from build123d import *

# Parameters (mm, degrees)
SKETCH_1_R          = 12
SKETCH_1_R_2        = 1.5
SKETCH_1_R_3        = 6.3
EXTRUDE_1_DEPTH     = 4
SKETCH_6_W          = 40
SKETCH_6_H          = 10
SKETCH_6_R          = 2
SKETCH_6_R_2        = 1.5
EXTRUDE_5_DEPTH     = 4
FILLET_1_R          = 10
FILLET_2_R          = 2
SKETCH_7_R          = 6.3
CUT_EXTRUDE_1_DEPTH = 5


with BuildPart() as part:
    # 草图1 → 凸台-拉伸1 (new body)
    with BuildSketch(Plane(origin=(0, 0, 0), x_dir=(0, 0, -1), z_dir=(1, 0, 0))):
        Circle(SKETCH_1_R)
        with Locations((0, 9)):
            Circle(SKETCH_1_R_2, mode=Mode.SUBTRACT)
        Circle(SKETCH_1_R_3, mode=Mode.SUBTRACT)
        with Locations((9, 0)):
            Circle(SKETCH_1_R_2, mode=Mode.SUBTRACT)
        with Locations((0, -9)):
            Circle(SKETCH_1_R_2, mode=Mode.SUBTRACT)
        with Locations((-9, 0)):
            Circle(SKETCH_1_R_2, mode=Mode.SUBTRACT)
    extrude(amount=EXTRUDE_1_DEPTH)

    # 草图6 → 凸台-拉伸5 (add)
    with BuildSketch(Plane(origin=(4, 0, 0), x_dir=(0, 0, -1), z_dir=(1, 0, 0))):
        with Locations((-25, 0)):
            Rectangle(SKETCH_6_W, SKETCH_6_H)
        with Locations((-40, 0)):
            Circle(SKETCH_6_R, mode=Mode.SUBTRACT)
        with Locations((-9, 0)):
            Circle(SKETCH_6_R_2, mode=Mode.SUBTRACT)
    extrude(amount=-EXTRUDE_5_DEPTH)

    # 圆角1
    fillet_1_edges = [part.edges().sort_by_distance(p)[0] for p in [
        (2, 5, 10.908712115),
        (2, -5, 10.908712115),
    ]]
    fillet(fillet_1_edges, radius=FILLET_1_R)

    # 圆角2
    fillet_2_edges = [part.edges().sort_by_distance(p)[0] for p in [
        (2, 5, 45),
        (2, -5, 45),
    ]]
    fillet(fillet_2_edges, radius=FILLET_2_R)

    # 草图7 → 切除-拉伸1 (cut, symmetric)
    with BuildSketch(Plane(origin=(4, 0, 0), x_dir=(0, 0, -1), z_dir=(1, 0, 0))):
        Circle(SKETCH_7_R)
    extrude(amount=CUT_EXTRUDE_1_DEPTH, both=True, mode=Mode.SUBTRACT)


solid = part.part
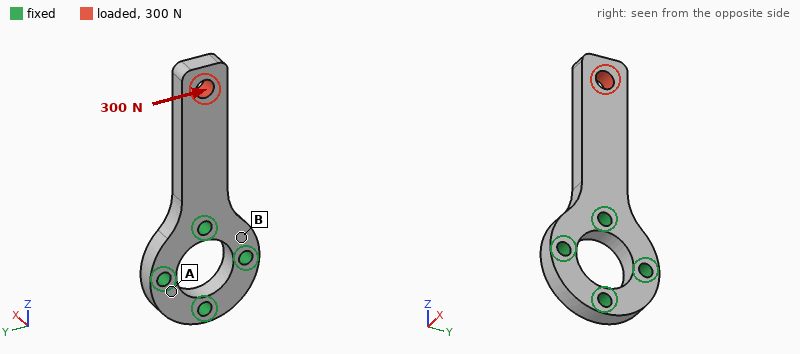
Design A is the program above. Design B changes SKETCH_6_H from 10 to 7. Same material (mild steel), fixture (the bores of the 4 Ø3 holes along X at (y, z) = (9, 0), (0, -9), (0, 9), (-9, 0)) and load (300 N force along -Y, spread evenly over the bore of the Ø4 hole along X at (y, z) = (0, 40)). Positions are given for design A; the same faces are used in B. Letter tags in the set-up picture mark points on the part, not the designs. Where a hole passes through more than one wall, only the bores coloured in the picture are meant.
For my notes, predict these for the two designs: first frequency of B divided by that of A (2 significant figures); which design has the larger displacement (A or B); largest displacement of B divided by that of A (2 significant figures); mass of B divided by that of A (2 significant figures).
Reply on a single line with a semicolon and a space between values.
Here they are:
1.1; B; 2.3; 0.84
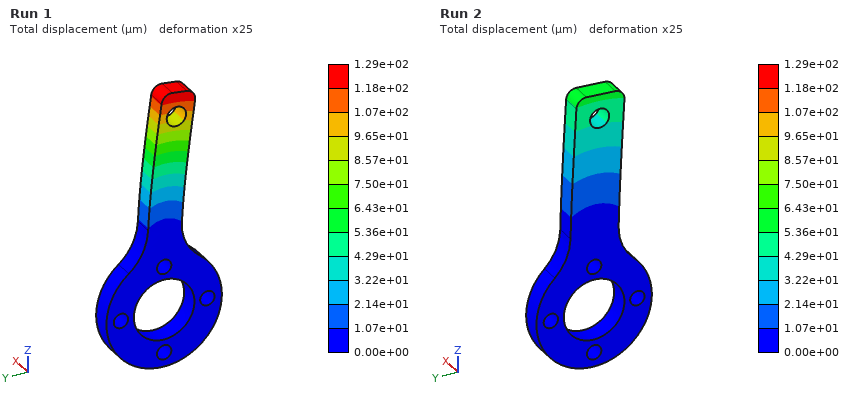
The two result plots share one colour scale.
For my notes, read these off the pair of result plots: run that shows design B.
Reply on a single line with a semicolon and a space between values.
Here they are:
Run 1
